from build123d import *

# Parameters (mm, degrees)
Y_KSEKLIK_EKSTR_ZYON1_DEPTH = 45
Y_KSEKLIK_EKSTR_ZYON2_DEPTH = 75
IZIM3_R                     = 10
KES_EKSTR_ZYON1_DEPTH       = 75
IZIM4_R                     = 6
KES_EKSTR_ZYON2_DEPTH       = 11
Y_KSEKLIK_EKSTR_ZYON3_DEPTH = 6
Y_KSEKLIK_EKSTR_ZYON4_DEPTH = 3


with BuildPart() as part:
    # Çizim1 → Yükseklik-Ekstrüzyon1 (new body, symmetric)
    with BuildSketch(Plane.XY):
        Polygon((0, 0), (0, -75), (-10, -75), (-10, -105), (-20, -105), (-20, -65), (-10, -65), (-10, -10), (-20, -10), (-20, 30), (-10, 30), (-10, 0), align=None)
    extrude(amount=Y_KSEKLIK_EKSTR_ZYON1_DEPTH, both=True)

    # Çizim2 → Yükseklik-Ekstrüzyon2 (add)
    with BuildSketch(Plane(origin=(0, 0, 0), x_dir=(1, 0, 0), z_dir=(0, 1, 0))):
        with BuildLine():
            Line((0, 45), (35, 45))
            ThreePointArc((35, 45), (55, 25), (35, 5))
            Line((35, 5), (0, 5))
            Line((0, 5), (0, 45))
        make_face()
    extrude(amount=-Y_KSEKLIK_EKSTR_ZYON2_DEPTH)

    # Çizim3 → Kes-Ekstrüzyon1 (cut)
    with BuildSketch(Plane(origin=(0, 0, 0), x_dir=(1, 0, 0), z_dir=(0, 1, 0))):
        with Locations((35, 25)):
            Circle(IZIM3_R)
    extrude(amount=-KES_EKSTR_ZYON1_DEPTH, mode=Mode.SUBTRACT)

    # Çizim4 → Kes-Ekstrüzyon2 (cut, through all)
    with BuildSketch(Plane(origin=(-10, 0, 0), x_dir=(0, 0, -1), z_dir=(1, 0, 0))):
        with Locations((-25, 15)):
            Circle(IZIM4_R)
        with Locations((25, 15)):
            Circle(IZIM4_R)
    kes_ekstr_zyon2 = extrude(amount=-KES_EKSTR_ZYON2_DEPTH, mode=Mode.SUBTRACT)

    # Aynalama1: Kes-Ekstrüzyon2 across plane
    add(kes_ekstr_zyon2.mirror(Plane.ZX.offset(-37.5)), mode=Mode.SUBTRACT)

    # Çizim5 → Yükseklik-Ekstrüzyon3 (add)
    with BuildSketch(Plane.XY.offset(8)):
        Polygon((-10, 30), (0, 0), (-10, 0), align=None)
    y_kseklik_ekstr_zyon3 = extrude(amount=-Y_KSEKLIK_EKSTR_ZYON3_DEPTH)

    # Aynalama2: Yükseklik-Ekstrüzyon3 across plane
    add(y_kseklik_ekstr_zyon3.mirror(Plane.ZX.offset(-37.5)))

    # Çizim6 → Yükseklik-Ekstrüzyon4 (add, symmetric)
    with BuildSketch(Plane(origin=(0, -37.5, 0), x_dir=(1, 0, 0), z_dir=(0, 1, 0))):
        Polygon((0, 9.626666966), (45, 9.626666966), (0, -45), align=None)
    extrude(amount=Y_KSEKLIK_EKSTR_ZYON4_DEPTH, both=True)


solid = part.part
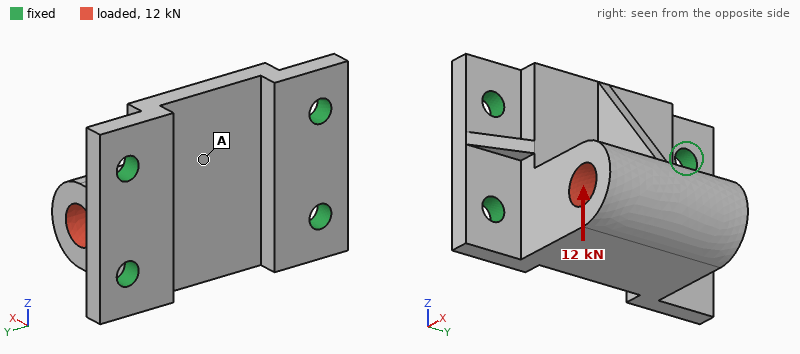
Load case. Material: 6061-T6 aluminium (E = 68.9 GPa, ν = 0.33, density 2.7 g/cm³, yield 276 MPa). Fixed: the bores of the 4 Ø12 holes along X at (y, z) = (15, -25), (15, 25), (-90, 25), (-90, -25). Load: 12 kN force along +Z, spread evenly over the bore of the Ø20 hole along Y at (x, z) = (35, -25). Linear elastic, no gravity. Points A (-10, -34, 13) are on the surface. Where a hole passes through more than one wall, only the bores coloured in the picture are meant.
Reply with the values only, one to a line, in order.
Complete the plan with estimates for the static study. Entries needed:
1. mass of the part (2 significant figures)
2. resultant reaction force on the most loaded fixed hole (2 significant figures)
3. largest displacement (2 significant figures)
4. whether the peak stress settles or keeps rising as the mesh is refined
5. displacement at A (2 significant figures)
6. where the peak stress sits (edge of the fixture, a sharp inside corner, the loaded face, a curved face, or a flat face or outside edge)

730 g
9.8 kN
0.17 mm
keeps rising
0.048 mm
edge of the fixture
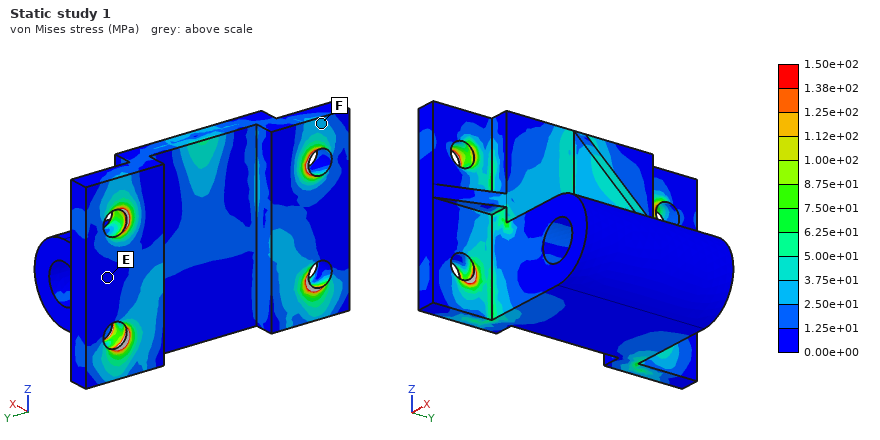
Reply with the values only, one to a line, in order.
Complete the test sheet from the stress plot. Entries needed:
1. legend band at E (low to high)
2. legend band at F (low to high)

0.00e+00 to 1.25e+01 MPa
2.50e+01 to 3.75e+01 MPa
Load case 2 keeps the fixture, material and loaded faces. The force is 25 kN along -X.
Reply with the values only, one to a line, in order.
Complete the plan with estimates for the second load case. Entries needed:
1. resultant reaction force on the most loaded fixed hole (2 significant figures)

14 kN
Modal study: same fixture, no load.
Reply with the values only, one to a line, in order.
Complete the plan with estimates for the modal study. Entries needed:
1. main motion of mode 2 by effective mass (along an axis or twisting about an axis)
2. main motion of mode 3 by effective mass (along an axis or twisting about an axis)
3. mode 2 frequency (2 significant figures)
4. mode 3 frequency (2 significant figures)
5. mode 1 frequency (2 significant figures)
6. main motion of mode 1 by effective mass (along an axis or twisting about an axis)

along Y
along X
5000 Hz
5200 Hz
2900 Hz
along Z
